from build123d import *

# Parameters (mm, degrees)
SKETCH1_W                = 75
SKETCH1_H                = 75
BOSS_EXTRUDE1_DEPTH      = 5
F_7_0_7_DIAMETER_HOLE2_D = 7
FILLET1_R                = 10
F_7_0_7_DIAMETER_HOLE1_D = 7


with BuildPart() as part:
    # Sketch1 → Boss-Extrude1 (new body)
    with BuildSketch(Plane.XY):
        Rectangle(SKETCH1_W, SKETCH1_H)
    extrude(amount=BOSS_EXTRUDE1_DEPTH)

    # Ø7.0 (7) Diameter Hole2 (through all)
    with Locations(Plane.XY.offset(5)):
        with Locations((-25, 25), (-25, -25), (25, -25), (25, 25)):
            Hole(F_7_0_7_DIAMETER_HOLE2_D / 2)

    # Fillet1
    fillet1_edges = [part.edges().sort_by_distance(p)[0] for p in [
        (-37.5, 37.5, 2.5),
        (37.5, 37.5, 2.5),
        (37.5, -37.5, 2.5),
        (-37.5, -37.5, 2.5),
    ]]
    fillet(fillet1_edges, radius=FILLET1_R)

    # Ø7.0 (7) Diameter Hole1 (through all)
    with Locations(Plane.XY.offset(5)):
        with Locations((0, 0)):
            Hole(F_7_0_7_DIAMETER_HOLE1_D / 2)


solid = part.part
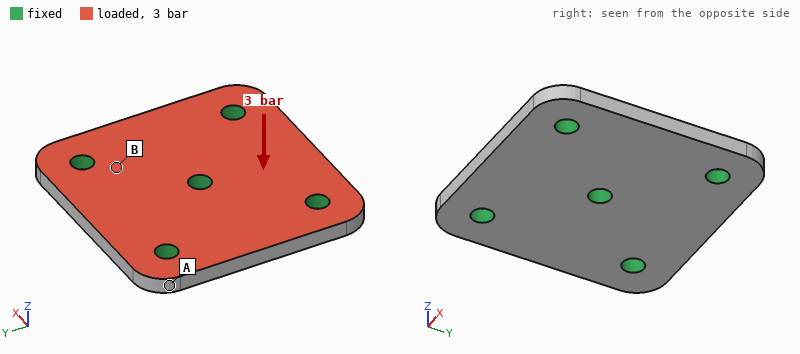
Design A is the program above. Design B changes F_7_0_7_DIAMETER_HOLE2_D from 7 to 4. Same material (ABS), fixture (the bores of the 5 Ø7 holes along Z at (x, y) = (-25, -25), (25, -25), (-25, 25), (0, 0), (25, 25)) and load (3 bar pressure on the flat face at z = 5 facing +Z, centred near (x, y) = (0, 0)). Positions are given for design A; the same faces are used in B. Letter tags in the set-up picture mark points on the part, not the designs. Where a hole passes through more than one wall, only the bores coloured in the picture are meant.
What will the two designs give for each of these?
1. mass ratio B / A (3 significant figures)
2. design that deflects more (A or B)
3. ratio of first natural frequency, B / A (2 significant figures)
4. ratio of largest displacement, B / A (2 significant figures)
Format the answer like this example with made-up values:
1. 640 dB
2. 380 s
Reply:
1. 1.02
2. B
3. 0.82
4. 1.2
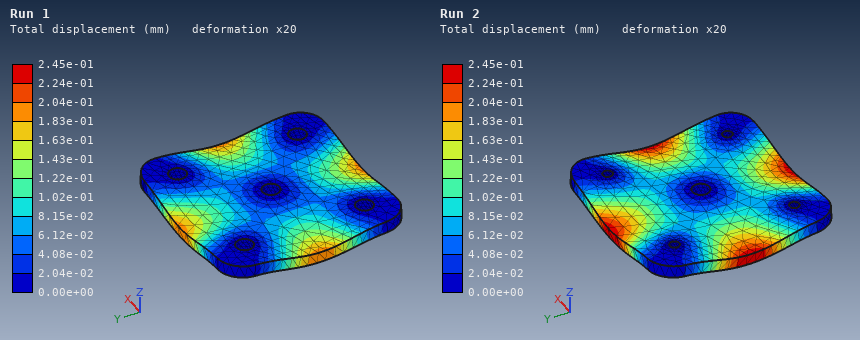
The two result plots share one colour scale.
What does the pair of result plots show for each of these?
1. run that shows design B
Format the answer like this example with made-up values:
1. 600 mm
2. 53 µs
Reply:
1. Run 2
